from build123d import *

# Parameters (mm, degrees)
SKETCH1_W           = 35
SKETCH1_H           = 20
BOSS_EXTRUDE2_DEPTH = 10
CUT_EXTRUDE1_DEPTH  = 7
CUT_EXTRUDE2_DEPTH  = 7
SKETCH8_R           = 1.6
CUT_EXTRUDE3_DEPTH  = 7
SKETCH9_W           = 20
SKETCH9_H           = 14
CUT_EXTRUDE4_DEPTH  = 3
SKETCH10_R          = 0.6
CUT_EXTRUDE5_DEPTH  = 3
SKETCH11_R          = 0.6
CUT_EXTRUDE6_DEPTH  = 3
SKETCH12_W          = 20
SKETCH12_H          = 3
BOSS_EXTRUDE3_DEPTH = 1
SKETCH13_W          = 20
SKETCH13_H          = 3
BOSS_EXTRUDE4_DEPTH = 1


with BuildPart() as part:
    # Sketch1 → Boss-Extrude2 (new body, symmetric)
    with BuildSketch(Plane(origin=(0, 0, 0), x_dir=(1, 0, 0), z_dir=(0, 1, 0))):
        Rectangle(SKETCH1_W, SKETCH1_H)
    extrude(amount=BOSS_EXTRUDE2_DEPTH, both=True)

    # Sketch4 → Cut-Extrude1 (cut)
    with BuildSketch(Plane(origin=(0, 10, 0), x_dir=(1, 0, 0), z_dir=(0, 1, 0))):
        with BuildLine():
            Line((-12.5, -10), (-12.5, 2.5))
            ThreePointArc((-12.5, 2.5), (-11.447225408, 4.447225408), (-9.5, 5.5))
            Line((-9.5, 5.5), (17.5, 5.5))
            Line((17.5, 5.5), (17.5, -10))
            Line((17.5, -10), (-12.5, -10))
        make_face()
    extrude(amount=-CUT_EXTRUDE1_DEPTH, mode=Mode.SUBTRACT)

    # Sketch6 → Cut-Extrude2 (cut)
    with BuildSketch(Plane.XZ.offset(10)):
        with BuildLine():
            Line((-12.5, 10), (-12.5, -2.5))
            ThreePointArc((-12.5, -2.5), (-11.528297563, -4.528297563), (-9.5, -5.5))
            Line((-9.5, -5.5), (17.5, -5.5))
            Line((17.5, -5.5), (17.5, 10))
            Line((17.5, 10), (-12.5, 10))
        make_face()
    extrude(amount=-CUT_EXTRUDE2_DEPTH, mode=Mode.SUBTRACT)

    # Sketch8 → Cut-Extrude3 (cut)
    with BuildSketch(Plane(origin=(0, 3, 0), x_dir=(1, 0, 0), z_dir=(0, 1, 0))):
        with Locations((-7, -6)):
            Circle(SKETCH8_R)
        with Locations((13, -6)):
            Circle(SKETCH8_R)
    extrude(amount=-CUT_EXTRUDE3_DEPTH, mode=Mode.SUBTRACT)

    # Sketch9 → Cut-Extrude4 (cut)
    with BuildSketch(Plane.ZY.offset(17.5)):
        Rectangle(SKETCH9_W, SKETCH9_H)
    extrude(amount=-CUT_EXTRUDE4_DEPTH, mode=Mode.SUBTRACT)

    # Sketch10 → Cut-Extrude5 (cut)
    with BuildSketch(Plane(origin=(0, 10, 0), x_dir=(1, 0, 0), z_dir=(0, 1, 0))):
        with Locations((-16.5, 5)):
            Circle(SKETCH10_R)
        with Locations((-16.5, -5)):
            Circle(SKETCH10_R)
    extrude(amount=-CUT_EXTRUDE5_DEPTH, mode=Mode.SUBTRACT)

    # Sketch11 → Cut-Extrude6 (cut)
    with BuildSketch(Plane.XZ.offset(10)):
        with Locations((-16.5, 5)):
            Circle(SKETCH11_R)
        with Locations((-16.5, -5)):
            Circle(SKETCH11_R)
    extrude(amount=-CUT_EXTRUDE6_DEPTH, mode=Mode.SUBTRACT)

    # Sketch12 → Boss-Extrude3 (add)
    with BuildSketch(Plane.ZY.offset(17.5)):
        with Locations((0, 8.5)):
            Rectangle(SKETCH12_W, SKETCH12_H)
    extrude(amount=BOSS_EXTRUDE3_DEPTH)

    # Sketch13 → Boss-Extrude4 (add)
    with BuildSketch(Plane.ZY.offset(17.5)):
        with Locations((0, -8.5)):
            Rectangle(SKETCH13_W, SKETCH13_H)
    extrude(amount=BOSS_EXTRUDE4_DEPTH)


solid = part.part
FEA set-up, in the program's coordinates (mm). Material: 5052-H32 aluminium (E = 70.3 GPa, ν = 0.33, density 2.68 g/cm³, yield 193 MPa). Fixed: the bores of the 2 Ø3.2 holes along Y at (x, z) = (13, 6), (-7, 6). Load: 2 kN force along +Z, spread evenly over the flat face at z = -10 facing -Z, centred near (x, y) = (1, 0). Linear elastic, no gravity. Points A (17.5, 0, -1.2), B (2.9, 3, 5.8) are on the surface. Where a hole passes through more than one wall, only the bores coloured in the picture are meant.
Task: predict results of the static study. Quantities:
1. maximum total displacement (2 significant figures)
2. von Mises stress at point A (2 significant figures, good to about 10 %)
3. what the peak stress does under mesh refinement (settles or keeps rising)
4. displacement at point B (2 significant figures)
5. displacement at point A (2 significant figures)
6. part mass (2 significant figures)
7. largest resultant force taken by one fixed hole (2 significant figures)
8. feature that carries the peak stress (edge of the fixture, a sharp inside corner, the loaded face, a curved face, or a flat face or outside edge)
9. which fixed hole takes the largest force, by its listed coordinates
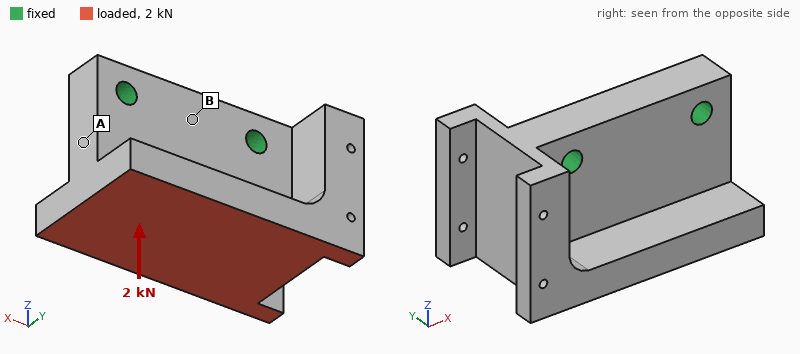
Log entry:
7.0 µm
8.1 MPa
keeps rising
1.7 µm
1.1 µm
18 g
1.2 kN
edge of the fixture
(-7, 6)
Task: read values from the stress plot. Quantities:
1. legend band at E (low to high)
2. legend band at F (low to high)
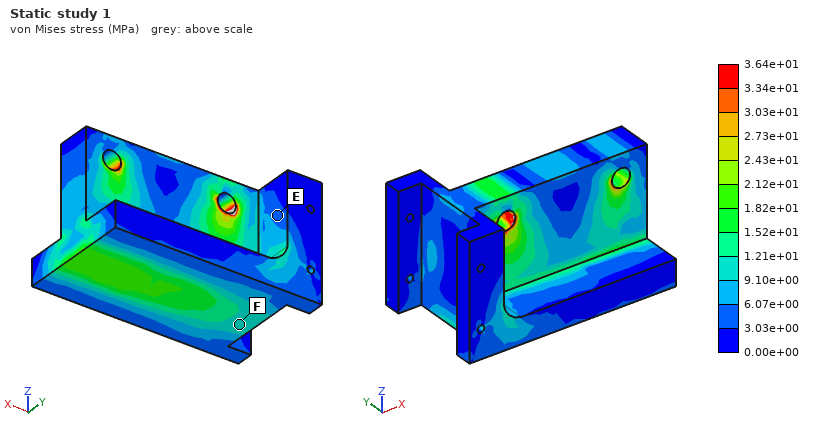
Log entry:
3.03e+00 to 6.07e+00 MPa
9.10e+00 to 1.21e+01 MPa
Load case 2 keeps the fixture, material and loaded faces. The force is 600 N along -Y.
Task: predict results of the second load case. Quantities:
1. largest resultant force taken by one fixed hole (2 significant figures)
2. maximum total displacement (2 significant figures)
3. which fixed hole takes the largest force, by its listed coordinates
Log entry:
360 N
30 µm
(-7, 6)
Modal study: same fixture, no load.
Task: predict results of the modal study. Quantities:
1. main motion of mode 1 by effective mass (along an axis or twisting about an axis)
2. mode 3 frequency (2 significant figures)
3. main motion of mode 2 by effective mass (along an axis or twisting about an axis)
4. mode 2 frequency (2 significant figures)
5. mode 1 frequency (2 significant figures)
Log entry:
along Y
20 kHz
twisting about Z
13 kHz
8600 Hz
